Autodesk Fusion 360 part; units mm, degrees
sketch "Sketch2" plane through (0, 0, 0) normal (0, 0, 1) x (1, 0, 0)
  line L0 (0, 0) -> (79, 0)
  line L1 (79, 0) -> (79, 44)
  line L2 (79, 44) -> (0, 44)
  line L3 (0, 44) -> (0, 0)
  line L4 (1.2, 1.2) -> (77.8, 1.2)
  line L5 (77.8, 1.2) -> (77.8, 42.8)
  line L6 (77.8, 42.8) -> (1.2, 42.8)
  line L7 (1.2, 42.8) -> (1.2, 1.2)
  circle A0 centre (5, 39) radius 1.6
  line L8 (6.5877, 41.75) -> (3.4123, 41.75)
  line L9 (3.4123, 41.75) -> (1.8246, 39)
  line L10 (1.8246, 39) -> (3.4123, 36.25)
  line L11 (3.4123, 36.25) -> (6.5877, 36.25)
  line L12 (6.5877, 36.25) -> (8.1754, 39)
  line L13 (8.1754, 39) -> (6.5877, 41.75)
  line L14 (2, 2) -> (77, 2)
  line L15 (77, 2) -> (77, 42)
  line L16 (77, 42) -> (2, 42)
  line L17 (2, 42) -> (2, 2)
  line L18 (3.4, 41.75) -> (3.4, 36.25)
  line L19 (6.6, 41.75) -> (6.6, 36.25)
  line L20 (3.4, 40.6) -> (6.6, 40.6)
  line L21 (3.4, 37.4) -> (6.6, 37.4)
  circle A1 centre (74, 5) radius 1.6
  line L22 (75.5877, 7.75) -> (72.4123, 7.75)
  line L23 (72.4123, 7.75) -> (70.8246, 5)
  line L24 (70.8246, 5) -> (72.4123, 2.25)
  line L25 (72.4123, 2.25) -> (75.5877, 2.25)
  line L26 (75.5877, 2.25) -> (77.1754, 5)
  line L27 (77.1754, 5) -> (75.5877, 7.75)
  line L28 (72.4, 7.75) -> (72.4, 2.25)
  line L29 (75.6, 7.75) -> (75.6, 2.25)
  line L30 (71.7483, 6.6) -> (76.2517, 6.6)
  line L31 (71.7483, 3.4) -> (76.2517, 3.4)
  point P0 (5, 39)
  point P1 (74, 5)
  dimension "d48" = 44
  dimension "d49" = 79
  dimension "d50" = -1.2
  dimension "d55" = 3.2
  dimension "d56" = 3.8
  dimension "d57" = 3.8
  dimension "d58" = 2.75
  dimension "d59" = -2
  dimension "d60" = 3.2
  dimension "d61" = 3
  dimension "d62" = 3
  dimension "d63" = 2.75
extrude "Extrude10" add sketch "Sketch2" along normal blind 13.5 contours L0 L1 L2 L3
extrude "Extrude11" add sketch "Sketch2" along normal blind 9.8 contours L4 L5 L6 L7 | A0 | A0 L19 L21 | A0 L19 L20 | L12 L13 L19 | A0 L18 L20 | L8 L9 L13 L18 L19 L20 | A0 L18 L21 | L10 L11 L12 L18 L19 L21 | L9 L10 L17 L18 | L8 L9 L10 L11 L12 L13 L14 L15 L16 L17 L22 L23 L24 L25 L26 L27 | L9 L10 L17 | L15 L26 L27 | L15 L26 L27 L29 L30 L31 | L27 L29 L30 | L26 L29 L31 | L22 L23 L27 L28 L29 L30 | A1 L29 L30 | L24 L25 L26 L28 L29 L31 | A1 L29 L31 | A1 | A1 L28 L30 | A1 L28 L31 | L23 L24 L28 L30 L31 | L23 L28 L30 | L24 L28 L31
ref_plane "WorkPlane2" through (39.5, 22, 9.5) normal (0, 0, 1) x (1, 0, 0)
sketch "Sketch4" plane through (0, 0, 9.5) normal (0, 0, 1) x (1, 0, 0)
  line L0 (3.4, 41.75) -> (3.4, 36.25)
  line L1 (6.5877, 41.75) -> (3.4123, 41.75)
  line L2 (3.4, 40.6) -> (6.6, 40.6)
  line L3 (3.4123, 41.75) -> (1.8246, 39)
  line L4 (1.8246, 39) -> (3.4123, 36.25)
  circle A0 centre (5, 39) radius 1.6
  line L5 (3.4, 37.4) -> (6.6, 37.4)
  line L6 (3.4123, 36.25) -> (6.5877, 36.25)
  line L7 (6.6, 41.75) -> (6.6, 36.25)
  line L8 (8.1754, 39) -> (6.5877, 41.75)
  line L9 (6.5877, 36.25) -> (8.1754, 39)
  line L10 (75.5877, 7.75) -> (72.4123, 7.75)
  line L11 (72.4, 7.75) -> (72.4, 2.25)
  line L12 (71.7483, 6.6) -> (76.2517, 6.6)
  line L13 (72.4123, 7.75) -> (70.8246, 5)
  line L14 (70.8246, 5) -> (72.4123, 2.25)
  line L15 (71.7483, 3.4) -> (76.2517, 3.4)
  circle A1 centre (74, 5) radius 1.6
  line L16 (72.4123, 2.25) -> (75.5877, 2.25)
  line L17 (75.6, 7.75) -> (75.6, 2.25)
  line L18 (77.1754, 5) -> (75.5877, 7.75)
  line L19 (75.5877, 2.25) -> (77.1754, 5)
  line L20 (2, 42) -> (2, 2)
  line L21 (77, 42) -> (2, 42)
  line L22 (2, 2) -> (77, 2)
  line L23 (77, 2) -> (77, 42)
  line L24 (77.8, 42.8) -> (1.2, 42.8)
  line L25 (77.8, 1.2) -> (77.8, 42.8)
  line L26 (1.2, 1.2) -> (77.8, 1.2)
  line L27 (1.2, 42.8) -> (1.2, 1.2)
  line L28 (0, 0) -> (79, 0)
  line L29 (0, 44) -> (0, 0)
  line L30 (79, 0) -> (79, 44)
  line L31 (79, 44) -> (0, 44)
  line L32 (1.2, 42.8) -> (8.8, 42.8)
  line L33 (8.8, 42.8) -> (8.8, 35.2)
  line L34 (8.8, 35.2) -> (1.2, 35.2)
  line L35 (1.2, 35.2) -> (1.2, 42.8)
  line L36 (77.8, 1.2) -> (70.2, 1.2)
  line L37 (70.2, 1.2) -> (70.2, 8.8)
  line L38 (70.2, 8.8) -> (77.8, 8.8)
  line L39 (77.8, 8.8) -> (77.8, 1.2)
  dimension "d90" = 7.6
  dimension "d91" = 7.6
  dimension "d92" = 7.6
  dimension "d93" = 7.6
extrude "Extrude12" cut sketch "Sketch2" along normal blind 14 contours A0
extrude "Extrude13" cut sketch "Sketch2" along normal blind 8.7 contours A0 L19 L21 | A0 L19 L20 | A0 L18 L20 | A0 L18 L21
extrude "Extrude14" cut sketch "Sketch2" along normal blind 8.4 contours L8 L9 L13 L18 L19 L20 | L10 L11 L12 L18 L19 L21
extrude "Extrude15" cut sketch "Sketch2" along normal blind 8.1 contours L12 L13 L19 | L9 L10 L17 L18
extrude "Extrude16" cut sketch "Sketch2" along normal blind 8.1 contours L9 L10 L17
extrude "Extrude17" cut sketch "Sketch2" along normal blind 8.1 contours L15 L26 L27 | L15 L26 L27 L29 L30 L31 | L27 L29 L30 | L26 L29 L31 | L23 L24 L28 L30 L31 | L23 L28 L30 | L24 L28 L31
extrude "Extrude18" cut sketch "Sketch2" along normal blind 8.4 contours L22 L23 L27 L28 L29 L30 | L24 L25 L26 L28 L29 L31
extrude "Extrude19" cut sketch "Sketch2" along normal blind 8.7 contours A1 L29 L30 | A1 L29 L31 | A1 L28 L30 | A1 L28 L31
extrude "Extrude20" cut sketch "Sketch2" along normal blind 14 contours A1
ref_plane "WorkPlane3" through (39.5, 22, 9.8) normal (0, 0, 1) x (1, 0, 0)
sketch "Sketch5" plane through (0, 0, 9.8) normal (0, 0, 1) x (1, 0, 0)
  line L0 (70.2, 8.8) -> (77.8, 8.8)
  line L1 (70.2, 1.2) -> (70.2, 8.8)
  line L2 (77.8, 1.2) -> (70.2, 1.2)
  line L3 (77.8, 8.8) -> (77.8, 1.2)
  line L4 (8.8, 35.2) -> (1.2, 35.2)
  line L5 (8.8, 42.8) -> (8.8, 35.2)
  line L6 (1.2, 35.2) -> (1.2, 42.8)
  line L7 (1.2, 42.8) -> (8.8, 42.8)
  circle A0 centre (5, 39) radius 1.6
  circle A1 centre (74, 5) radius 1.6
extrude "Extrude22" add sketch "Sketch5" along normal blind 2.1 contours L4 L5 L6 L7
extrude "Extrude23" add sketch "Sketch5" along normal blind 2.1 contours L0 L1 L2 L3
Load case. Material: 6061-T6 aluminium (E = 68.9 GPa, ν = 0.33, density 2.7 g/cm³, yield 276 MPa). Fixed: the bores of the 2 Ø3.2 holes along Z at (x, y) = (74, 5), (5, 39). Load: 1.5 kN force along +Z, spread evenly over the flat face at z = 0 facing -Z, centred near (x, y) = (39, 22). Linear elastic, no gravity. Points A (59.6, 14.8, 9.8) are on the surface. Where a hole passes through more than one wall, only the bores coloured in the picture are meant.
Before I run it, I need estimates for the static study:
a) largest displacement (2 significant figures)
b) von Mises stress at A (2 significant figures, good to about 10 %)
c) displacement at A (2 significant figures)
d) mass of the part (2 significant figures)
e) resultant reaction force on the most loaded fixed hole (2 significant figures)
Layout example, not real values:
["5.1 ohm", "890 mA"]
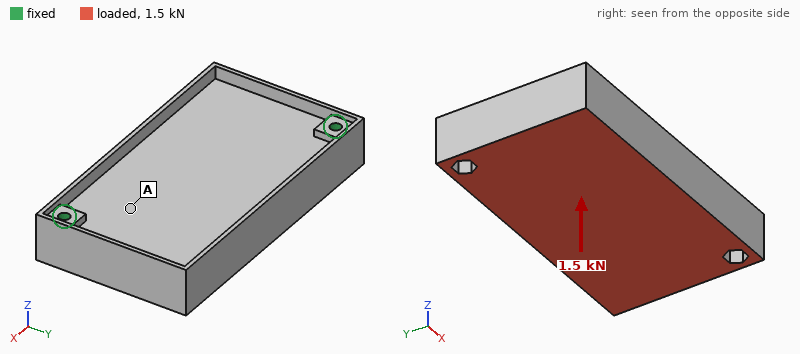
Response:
["33 µm", "7.7 MPa", "17 µm", "94 g", "1.2 kN"]
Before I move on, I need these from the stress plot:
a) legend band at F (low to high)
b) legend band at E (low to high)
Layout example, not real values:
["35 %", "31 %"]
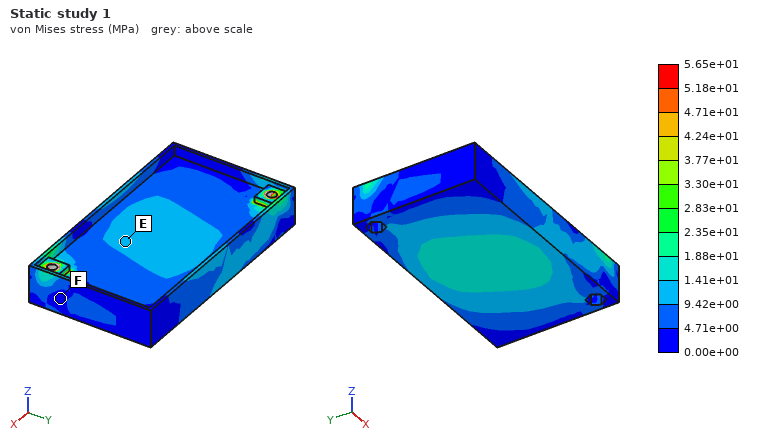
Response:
["0.00e+00 to 4.71e+00 MPa", "9.42e+00 to 1.41e+01 MPa"]
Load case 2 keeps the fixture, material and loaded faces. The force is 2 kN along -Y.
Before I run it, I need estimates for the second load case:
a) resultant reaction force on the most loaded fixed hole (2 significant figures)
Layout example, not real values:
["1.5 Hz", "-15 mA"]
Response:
["1.0 kN"]
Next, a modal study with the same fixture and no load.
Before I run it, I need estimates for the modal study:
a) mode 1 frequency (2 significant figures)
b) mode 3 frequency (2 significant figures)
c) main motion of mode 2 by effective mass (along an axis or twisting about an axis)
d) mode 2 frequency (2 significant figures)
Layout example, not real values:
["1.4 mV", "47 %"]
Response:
["1900 Hz", "8200 Hz", "along Z", "4100 Hz"]
